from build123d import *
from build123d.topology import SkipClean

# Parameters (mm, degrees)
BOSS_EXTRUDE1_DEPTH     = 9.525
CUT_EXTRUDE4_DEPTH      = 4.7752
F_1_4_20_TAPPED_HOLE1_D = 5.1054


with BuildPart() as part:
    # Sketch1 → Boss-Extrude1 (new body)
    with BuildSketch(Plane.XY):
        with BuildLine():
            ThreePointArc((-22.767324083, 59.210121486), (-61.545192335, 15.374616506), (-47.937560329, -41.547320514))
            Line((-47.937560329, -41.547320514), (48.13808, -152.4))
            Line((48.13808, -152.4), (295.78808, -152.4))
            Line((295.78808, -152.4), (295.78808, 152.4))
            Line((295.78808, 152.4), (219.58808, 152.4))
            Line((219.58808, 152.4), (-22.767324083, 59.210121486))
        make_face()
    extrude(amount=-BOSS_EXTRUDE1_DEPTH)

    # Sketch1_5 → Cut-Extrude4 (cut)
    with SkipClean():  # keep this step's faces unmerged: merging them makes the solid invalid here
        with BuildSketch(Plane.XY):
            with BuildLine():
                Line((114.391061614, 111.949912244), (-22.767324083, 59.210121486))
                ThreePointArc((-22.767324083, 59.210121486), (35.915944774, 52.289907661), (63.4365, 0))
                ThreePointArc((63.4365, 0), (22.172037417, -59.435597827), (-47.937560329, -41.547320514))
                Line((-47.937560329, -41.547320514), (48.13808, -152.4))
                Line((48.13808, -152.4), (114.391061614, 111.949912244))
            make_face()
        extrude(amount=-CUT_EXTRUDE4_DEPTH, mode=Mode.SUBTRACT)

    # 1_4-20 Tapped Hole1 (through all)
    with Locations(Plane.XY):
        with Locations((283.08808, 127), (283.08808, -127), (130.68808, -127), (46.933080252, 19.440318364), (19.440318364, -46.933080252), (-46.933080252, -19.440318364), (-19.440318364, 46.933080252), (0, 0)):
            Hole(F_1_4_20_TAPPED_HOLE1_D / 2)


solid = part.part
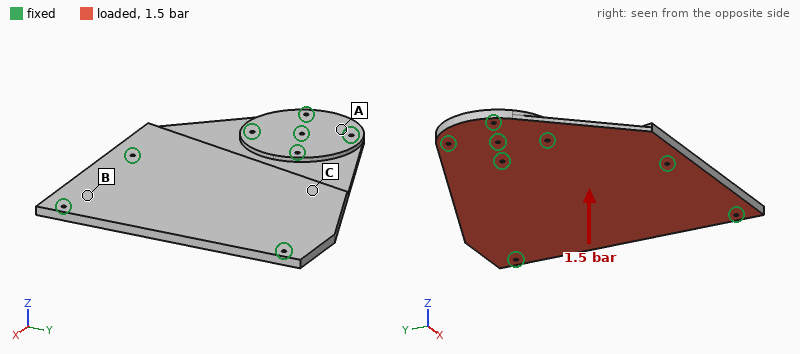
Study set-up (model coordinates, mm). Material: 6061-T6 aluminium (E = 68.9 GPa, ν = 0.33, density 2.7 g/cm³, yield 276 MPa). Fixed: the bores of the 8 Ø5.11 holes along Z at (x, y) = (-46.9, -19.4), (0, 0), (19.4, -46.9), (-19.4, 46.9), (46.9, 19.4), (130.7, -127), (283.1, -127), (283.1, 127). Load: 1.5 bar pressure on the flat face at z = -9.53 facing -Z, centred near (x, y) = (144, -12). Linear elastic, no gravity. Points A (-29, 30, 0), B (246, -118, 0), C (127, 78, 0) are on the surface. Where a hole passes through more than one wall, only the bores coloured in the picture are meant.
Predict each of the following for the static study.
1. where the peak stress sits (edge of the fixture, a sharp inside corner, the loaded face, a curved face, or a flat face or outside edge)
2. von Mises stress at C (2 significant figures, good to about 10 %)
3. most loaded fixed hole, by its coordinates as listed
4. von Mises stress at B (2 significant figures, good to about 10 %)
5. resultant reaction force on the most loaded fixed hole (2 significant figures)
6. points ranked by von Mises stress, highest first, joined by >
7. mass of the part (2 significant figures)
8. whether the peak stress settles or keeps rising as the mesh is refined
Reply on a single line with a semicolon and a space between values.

edge of the fixture; 38 MPa; (46.9, 19.4); 21 MPa; 3.8 kN; C > B > A; 2.1 kg; keeps rising
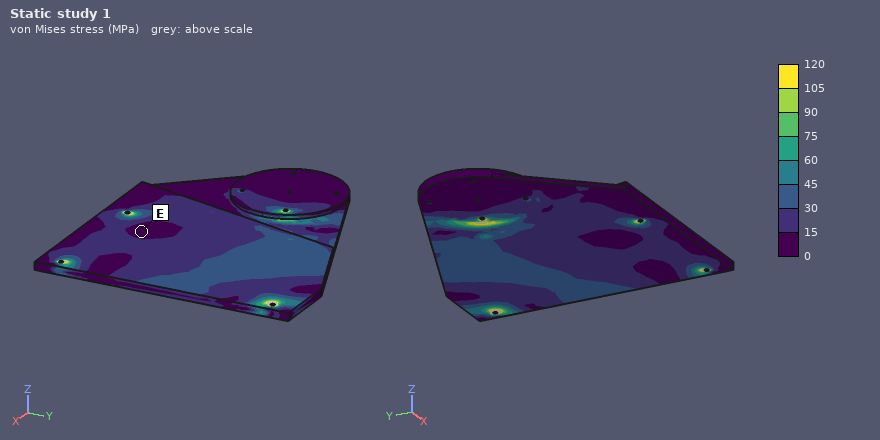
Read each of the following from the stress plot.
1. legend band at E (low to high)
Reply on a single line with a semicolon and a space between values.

0 to 15 MPa
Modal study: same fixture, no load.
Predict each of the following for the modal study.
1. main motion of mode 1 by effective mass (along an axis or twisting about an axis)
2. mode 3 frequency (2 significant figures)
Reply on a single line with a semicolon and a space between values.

along Z; 1300 Hz
